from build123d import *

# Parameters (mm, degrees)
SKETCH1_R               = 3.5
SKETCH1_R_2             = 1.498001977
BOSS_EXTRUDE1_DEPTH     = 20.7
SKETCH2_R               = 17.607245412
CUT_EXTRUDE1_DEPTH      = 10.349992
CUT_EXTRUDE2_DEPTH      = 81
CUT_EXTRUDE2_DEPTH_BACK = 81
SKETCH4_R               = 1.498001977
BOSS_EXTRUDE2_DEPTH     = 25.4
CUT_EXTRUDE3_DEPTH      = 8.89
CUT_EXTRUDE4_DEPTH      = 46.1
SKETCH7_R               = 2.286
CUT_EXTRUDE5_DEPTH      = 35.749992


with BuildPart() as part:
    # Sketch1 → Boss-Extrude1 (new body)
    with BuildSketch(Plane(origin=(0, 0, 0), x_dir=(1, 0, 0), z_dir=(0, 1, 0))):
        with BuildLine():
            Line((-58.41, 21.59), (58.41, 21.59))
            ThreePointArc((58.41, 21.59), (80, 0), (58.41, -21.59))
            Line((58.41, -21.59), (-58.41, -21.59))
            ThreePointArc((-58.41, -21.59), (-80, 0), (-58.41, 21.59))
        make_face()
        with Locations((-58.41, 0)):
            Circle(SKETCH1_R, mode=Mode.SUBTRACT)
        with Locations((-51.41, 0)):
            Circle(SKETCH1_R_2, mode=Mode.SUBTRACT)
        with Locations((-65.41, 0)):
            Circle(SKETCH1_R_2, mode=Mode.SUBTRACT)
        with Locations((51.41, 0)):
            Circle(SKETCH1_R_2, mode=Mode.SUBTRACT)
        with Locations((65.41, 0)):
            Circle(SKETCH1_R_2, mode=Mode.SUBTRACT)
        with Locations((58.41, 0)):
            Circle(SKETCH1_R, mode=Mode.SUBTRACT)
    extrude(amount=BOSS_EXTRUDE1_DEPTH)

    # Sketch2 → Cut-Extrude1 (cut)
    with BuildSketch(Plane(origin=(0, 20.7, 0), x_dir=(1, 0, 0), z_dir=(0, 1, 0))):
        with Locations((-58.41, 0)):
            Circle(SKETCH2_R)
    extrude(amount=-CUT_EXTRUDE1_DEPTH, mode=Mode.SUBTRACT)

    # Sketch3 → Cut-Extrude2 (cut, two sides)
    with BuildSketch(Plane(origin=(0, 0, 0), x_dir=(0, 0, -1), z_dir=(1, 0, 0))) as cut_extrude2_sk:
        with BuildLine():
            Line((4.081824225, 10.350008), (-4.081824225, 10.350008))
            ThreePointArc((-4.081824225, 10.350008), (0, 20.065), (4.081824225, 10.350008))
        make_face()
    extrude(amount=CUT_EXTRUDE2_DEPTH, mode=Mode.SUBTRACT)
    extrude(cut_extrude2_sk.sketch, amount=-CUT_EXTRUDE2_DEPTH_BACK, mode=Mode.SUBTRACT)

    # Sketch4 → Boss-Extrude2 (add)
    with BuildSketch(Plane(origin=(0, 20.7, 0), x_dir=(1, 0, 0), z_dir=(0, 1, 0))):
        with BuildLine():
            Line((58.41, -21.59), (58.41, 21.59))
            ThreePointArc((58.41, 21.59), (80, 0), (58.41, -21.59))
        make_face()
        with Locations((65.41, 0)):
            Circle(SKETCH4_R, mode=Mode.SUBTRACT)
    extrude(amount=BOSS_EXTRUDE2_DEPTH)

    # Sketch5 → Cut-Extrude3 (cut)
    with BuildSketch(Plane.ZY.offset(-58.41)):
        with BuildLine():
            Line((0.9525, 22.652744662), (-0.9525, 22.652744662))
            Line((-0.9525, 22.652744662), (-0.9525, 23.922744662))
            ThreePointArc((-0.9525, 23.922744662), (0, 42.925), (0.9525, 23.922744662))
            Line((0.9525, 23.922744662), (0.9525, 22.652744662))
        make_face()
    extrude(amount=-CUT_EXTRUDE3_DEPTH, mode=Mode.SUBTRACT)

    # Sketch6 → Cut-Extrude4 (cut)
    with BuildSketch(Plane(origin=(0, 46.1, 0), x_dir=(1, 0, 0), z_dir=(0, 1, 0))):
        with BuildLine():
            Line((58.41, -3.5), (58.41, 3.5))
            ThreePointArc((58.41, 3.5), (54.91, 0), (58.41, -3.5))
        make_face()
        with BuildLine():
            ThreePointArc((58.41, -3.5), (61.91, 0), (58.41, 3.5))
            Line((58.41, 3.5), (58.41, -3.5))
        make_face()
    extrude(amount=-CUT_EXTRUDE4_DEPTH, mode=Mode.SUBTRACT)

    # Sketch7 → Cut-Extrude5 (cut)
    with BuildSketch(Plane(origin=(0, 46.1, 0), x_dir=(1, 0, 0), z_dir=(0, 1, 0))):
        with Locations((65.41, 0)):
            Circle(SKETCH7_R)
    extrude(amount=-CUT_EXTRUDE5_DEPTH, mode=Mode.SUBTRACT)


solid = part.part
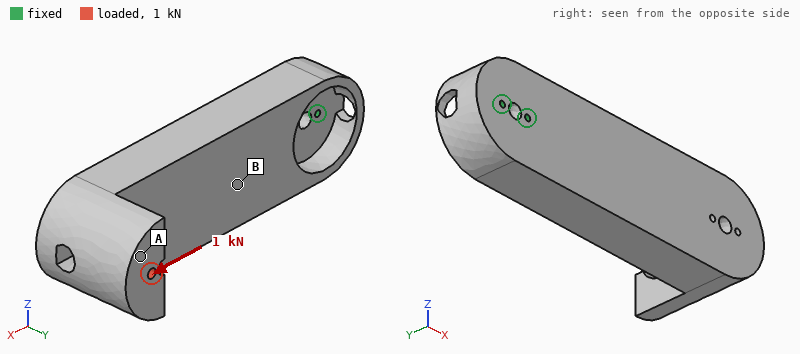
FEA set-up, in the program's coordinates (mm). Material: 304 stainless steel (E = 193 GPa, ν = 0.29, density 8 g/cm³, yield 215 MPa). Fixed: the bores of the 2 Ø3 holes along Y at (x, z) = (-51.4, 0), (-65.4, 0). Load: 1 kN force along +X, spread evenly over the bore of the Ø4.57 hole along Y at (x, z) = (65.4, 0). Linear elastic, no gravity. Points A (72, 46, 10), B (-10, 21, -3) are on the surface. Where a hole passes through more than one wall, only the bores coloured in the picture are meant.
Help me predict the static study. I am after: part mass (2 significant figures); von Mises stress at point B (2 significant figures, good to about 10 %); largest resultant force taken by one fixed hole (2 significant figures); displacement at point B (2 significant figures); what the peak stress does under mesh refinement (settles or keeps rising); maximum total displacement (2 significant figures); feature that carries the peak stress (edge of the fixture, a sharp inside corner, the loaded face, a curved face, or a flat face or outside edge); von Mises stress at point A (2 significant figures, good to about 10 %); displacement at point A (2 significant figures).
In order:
1.0 kg
9.4 MPa
1.2 kN
16 µm
keeps rising
79 µm
edge of the fixture
3.0 MPa
72 µm
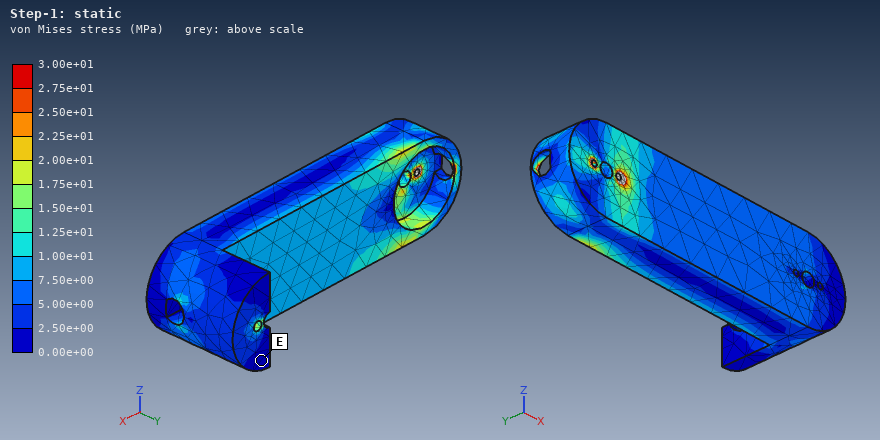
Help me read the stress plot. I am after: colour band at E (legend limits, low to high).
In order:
0.00e+00 to 2.50e+00 MPa
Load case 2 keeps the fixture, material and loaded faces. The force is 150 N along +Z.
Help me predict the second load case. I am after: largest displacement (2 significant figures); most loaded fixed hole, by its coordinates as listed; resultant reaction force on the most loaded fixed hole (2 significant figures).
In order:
19 µm
(-51.4, 0)
1.2 kN
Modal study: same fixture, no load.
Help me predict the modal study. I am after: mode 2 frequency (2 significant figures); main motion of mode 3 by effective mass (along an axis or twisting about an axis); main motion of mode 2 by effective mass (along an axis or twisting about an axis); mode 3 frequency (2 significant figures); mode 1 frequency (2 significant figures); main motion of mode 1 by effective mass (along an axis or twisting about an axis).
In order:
810 Hz
twisting about X
along Z
2000 Hz
500 Hz
along Y
